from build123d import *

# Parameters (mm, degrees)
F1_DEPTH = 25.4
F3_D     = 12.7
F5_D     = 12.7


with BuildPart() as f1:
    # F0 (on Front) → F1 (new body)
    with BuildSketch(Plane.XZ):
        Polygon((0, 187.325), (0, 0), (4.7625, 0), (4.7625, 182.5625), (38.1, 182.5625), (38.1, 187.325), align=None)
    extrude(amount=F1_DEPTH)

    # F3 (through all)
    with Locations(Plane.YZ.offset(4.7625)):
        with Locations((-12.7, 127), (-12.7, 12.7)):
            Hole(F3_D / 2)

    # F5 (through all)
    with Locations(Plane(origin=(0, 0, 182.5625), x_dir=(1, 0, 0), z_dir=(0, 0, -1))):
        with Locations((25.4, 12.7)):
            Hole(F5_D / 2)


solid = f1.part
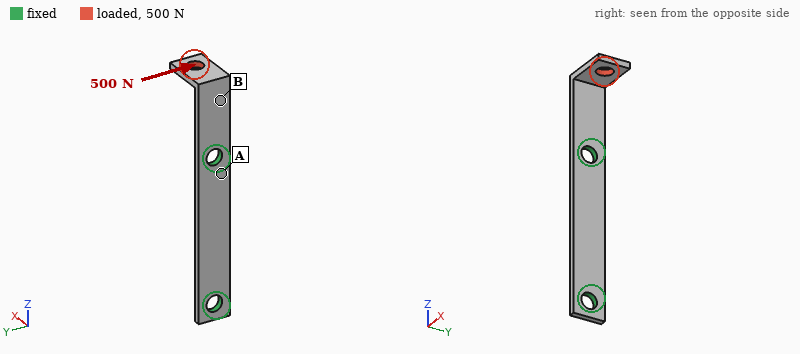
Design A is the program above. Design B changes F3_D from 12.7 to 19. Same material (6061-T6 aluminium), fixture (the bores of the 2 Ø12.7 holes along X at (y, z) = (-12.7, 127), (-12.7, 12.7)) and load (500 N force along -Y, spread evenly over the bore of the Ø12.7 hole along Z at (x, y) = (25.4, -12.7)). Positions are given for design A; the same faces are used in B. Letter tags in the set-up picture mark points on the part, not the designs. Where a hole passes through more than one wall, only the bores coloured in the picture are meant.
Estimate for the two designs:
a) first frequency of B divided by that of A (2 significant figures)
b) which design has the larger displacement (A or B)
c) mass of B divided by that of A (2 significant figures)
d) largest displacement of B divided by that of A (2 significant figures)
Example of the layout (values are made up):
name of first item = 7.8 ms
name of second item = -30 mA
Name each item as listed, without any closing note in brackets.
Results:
first frequency of B divided by that of A = 1.1
which design has the larger displacement = A
mass of B divided by that of A = 0.94
largest displacement of B divided by that of A = 0.90
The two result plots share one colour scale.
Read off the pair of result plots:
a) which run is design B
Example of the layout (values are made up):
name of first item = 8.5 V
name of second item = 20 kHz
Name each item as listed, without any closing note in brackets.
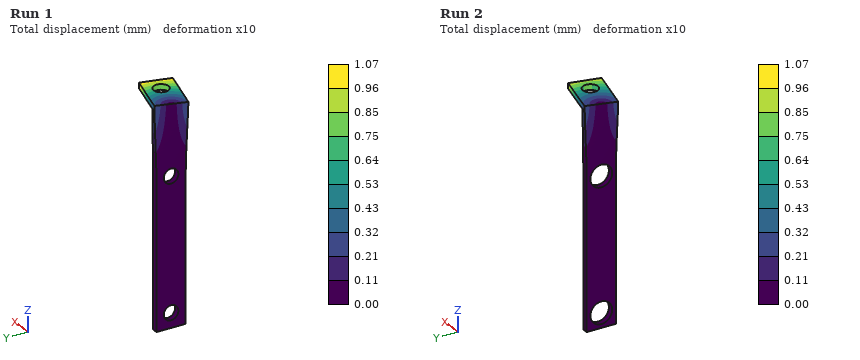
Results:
which run is design B = Run 2
